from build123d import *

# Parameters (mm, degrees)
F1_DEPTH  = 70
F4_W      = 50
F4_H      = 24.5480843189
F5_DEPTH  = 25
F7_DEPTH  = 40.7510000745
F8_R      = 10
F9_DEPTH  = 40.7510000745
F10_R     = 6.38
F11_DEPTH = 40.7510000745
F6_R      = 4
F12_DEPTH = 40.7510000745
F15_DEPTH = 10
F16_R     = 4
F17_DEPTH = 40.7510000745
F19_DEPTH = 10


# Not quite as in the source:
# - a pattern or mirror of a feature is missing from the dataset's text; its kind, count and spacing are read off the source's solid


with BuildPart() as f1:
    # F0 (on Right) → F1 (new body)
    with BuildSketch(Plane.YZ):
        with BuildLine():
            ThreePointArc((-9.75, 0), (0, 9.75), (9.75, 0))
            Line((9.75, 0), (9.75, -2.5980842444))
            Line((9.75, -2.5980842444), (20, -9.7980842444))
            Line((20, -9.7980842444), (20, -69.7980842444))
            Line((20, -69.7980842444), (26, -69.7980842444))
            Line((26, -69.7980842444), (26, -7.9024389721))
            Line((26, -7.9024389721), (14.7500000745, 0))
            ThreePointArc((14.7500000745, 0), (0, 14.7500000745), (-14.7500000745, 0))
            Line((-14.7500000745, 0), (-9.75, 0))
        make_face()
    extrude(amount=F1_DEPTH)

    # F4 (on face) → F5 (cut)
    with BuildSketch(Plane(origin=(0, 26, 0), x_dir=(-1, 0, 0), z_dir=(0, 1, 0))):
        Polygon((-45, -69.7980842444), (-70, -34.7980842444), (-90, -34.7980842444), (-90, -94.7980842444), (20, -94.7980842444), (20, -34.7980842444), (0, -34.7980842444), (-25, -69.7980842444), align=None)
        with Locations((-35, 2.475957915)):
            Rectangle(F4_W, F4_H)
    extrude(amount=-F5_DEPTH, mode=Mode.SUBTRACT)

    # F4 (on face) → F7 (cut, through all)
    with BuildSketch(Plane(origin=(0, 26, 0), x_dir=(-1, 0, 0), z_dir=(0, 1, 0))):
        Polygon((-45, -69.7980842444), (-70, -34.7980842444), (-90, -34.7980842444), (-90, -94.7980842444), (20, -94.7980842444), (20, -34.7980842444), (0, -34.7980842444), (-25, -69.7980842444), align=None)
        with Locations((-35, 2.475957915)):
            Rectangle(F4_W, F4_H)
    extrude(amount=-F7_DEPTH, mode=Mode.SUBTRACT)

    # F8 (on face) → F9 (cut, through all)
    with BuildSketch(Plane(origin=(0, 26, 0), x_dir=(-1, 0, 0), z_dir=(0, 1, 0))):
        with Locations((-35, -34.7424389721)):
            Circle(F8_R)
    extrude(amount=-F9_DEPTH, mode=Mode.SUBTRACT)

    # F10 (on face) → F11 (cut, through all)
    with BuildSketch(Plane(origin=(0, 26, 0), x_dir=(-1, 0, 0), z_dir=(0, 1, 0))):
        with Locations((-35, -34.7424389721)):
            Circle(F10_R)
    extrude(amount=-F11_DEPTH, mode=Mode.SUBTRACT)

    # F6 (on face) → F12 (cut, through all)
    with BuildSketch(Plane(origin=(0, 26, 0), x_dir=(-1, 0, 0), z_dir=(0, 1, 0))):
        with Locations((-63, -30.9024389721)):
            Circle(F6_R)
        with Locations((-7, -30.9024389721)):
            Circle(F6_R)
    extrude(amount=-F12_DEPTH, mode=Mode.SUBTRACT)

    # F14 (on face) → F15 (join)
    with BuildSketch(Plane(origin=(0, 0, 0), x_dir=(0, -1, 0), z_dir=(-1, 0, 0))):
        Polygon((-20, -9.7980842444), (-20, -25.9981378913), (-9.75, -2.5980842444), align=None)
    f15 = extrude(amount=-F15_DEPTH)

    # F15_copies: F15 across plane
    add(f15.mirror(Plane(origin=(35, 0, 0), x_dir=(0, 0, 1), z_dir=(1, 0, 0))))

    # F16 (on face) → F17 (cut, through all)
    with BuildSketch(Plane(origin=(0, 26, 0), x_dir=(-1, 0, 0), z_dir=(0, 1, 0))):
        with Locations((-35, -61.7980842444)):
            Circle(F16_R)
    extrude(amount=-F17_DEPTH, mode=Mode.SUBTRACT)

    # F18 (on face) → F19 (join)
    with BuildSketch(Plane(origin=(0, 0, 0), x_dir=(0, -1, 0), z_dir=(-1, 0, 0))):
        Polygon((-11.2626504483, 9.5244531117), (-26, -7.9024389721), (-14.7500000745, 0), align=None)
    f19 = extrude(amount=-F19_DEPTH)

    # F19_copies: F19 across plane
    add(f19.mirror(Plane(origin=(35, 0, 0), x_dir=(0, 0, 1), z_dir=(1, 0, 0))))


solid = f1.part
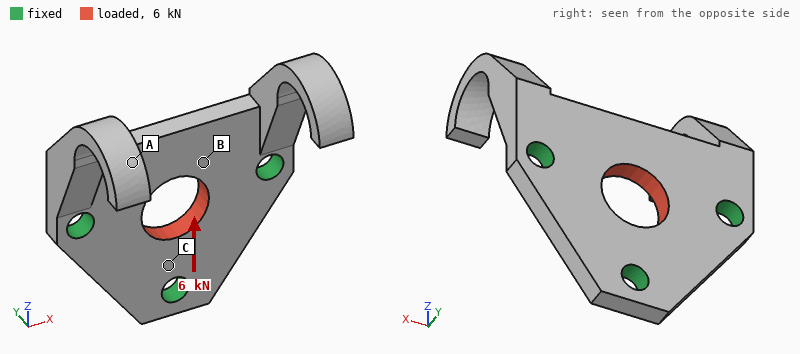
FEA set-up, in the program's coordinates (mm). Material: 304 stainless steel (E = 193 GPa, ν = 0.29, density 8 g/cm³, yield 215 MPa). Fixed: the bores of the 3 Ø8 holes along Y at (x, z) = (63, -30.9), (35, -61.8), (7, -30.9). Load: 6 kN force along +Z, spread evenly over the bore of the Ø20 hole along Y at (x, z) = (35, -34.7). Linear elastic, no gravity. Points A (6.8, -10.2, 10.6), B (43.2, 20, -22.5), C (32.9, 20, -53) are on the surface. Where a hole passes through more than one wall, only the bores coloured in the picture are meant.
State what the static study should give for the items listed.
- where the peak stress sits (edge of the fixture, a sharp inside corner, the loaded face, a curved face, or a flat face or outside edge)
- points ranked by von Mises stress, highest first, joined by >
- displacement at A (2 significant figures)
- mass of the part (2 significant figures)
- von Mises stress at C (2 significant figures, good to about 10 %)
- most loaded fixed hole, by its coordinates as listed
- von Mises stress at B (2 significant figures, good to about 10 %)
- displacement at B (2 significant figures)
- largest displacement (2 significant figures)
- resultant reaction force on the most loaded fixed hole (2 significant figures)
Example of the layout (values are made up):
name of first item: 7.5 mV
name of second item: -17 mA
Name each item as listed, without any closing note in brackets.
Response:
where the peak stress sits: edge of the fixture
points ranked by von Mises stress, highest first, joined by >: C > B > A
displacement at A: 3.8 µm
mass of the part: 200 g
von Mises stress at C: 28 MPa
most loaded fixed hole, by its coordinates as listed: (35, -61.8)
von Mises stress at B: 18 MPa
displacement at B: 3.6 µm
largest displacement: 4.7 µm
resultant reaction force on the most loaded fixed hole: 2.5 kN
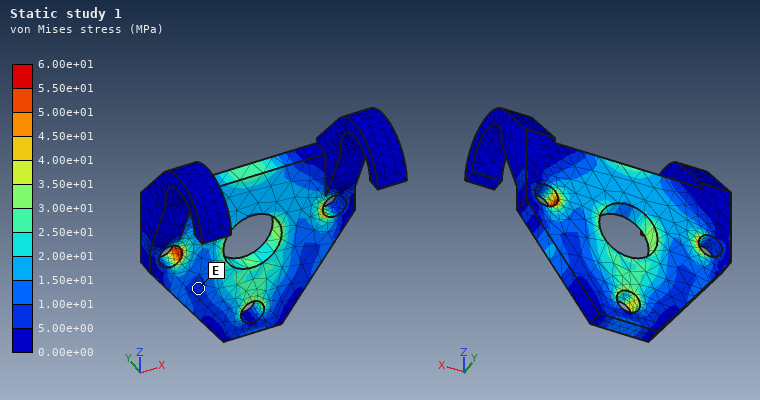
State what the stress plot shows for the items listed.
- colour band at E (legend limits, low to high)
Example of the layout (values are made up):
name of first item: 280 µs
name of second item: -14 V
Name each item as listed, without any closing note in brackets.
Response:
colour band at E: 5.00e+00 to 1.00e+01 MPa
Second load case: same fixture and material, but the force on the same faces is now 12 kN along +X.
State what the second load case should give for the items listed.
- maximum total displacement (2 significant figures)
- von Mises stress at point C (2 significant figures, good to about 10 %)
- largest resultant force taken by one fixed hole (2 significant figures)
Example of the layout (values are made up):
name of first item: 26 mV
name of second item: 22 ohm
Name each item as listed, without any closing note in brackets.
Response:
maximum total displacement: 5.5 µm
von Mises stress at point C: 19 MPa
largest resultant force taken by one fixed hole: 4.8 kN
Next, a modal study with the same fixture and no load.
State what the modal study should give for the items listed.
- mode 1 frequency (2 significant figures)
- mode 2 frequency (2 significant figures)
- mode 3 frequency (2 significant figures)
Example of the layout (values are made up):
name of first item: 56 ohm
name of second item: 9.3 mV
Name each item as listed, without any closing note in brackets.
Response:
mode 1 frequency: 2100 Hz
mode 2 frequency: 2200 Hz
mode 3 frequency: 2700 Hz
